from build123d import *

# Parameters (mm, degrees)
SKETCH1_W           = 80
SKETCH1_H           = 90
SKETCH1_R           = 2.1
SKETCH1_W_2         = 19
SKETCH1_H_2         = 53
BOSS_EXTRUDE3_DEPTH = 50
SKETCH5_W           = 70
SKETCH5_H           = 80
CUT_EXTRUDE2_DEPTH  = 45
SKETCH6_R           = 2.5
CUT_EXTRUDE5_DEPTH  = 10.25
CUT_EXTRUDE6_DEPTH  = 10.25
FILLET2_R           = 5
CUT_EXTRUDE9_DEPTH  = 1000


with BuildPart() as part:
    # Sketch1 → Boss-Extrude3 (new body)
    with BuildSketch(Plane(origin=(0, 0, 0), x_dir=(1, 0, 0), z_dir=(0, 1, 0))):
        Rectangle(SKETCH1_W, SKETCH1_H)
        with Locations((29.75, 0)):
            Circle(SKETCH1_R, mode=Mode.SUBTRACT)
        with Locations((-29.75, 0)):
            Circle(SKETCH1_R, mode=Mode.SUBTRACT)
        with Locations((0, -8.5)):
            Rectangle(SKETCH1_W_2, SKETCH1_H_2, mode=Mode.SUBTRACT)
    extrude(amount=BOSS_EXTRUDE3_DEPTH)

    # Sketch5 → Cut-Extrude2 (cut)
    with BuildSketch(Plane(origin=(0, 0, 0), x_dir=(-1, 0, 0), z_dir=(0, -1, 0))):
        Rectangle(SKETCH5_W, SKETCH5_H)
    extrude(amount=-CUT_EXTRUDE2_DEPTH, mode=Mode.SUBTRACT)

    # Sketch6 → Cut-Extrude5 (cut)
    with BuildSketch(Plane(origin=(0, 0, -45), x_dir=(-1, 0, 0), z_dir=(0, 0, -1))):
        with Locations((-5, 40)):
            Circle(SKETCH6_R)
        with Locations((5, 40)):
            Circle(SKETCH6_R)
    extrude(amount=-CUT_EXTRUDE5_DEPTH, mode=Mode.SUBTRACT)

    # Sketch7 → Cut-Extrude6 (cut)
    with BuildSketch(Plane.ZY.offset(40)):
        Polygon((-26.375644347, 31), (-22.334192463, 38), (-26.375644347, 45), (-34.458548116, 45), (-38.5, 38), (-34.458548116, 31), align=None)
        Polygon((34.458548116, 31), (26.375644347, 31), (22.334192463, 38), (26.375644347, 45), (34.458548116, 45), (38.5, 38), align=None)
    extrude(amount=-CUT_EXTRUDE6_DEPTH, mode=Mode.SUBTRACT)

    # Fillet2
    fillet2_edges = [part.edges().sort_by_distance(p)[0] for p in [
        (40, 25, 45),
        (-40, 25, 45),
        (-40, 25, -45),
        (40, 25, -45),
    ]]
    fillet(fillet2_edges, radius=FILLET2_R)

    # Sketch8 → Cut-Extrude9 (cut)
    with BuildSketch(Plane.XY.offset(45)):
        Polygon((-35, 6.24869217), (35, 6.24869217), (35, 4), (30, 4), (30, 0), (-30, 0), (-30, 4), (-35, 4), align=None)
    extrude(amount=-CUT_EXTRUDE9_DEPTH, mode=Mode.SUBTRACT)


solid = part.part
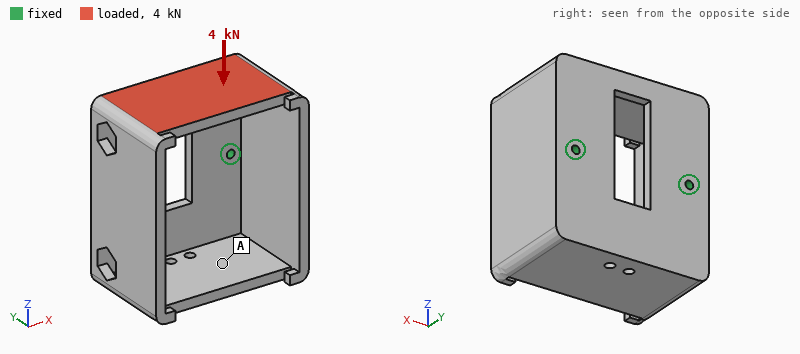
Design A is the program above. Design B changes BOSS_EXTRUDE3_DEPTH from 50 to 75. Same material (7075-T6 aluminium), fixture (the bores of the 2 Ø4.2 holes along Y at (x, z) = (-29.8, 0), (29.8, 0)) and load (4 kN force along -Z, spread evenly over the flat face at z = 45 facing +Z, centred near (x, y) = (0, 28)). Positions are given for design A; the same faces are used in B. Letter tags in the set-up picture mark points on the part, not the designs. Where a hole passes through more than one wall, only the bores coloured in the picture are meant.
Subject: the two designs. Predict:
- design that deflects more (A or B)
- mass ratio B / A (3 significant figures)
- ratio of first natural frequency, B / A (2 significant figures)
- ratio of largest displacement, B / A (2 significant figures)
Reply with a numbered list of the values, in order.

1. A
2. 2.60
3. 4.3
4. 0.18
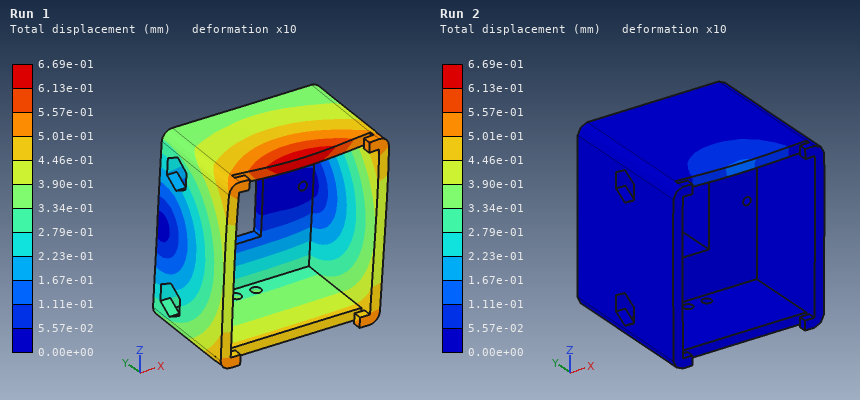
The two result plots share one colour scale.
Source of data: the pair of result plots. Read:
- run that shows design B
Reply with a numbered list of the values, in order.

1. Run 2
